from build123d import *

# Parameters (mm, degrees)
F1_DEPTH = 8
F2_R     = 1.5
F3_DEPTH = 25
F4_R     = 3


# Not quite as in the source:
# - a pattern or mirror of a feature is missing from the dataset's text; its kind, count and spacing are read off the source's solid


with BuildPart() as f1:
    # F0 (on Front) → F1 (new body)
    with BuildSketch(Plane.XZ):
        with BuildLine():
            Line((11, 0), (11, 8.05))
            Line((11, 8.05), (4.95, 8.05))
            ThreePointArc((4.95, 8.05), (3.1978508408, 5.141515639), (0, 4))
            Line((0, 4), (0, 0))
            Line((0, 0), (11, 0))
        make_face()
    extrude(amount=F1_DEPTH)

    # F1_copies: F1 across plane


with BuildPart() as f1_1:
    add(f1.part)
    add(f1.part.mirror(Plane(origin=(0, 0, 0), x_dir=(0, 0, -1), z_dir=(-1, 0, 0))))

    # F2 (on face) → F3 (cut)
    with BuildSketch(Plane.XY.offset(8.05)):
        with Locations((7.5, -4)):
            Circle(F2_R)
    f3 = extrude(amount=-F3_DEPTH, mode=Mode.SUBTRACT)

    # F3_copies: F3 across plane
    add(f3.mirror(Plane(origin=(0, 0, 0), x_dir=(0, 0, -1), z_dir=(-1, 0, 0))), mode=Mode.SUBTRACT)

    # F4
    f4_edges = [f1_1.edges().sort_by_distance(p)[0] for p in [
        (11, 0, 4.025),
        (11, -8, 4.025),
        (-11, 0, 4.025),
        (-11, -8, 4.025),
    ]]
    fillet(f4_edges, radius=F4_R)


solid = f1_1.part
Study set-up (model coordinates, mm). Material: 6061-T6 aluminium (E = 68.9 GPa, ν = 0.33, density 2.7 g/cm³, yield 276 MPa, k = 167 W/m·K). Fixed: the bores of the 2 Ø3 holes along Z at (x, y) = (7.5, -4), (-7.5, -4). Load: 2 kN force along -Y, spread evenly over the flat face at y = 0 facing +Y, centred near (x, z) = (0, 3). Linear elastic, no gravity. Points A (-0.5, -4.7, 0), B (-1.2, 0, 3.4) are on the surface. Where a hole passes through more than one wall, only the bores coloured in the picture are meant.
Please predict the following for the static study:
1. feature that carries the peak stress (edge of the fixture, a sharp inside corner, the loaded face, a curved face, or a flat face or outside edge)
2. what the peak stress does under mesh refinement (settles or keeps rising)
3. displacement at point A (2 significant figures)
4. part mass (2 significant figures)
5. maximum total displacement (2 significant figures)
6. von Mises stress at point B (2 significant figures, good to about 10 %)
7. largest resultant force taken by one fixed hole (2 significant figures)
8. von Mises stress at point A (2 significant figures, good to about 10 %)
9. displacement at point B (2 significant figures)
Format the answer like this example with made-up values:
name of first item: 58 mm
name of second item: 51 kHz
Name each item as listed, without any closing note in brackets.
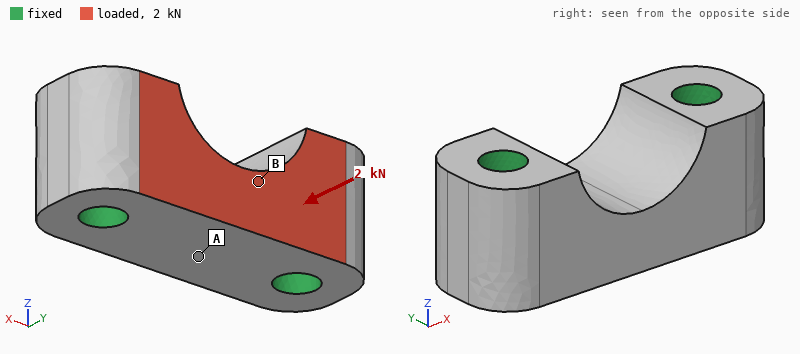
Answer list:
feature that carries the peak stress: edge of the fixture
what the peak stress does under mesh refinement: keeps rising
displacement at point A: 3.7 µm
part mass: 2.7 g
maximum total displacement: 4.8 µm
von Mises stress at point B: 29 MPa
largest resultant force taken by one fixed hole: 1.0 kN
von Mises stress at point A: 9.3 MPa
displacement at point B: 3.7 µm
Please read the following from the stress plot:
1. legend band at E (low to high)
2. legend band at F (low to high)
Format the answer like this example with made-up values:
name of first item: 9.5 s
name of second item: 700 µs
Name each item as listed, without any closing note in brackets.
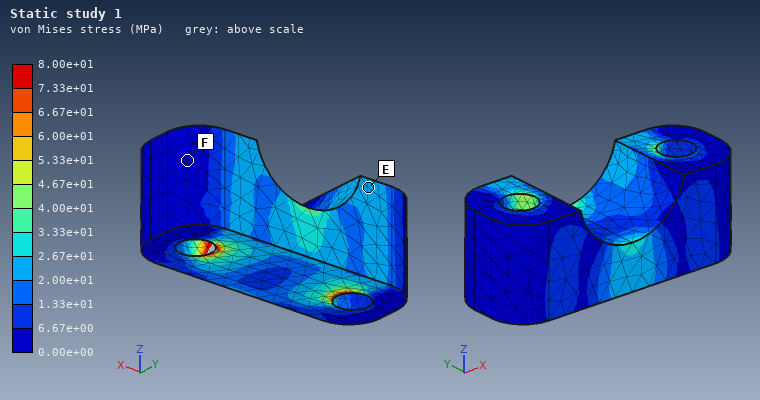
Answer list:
legend band at E: 2.00e+01 to 2.67e+01 MPa
legend band at F: 0.00e+00 to 6.67e+00 MPa
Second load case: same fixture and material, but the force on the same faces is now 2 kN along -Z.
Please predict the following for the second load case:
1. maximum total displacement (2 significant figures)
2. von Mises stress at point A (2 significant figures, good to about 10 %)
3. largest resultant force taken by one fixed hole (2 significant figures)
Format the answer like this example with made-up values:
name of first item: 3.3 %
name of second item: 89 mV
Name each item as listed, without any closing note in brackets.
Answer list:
maximum total displacement: 11 µm
von Mises stress at point A: 23 MPa
largest resultant force taken by one fixed hole: 1.0 kN
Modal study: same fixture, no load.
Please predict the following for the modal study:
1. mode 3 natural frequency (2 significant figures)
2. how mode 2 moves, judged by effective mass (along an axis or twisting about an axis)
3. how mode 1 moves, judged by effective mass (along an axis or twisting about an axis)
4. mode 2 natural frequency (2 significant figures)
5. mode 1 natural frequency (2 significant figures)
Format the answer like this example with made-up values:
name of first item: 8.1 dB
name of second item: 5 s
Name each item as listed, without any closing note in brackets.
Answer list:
mode 3 natural frequency: 130 kHz
how mode 2 moves, judged by effective mass: along Z
how mode 1 moves, judged by effective mass: along Y
mode 2 natural frequency: 100 kHz
mode 1 natural frequency: 92 kHz
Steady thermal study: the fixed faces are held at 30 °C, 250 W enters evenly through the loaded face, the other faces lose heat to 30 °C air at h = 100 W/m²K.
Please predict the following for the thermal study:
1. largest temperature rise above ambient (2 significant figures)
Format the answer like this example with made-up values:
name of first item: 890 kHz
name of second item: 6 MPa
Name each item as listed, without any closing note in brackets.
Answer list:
largest temperature rise above ambient: 81 K
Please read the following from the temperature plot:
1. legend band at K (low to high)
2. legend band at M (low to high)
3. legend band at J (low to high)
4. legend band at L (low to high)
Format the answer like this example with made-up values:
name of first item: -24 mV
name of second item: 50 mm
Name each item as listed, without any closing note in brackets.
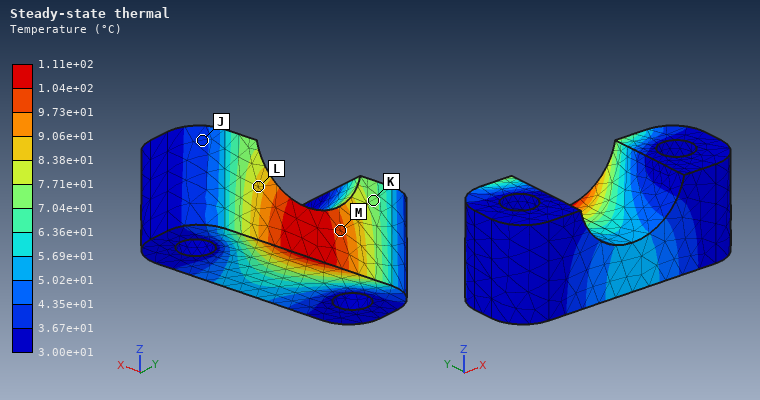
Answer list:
legend band at K: 7.04e+01 to 7.71e+01 °C
legend band at M: 9.73e+01 to 1.04e+02 °C
legend band at J: 3.67e+01 to 4.35e+01 °C
legend band at L: 8.38e+01 to 9.06e+01 °C
